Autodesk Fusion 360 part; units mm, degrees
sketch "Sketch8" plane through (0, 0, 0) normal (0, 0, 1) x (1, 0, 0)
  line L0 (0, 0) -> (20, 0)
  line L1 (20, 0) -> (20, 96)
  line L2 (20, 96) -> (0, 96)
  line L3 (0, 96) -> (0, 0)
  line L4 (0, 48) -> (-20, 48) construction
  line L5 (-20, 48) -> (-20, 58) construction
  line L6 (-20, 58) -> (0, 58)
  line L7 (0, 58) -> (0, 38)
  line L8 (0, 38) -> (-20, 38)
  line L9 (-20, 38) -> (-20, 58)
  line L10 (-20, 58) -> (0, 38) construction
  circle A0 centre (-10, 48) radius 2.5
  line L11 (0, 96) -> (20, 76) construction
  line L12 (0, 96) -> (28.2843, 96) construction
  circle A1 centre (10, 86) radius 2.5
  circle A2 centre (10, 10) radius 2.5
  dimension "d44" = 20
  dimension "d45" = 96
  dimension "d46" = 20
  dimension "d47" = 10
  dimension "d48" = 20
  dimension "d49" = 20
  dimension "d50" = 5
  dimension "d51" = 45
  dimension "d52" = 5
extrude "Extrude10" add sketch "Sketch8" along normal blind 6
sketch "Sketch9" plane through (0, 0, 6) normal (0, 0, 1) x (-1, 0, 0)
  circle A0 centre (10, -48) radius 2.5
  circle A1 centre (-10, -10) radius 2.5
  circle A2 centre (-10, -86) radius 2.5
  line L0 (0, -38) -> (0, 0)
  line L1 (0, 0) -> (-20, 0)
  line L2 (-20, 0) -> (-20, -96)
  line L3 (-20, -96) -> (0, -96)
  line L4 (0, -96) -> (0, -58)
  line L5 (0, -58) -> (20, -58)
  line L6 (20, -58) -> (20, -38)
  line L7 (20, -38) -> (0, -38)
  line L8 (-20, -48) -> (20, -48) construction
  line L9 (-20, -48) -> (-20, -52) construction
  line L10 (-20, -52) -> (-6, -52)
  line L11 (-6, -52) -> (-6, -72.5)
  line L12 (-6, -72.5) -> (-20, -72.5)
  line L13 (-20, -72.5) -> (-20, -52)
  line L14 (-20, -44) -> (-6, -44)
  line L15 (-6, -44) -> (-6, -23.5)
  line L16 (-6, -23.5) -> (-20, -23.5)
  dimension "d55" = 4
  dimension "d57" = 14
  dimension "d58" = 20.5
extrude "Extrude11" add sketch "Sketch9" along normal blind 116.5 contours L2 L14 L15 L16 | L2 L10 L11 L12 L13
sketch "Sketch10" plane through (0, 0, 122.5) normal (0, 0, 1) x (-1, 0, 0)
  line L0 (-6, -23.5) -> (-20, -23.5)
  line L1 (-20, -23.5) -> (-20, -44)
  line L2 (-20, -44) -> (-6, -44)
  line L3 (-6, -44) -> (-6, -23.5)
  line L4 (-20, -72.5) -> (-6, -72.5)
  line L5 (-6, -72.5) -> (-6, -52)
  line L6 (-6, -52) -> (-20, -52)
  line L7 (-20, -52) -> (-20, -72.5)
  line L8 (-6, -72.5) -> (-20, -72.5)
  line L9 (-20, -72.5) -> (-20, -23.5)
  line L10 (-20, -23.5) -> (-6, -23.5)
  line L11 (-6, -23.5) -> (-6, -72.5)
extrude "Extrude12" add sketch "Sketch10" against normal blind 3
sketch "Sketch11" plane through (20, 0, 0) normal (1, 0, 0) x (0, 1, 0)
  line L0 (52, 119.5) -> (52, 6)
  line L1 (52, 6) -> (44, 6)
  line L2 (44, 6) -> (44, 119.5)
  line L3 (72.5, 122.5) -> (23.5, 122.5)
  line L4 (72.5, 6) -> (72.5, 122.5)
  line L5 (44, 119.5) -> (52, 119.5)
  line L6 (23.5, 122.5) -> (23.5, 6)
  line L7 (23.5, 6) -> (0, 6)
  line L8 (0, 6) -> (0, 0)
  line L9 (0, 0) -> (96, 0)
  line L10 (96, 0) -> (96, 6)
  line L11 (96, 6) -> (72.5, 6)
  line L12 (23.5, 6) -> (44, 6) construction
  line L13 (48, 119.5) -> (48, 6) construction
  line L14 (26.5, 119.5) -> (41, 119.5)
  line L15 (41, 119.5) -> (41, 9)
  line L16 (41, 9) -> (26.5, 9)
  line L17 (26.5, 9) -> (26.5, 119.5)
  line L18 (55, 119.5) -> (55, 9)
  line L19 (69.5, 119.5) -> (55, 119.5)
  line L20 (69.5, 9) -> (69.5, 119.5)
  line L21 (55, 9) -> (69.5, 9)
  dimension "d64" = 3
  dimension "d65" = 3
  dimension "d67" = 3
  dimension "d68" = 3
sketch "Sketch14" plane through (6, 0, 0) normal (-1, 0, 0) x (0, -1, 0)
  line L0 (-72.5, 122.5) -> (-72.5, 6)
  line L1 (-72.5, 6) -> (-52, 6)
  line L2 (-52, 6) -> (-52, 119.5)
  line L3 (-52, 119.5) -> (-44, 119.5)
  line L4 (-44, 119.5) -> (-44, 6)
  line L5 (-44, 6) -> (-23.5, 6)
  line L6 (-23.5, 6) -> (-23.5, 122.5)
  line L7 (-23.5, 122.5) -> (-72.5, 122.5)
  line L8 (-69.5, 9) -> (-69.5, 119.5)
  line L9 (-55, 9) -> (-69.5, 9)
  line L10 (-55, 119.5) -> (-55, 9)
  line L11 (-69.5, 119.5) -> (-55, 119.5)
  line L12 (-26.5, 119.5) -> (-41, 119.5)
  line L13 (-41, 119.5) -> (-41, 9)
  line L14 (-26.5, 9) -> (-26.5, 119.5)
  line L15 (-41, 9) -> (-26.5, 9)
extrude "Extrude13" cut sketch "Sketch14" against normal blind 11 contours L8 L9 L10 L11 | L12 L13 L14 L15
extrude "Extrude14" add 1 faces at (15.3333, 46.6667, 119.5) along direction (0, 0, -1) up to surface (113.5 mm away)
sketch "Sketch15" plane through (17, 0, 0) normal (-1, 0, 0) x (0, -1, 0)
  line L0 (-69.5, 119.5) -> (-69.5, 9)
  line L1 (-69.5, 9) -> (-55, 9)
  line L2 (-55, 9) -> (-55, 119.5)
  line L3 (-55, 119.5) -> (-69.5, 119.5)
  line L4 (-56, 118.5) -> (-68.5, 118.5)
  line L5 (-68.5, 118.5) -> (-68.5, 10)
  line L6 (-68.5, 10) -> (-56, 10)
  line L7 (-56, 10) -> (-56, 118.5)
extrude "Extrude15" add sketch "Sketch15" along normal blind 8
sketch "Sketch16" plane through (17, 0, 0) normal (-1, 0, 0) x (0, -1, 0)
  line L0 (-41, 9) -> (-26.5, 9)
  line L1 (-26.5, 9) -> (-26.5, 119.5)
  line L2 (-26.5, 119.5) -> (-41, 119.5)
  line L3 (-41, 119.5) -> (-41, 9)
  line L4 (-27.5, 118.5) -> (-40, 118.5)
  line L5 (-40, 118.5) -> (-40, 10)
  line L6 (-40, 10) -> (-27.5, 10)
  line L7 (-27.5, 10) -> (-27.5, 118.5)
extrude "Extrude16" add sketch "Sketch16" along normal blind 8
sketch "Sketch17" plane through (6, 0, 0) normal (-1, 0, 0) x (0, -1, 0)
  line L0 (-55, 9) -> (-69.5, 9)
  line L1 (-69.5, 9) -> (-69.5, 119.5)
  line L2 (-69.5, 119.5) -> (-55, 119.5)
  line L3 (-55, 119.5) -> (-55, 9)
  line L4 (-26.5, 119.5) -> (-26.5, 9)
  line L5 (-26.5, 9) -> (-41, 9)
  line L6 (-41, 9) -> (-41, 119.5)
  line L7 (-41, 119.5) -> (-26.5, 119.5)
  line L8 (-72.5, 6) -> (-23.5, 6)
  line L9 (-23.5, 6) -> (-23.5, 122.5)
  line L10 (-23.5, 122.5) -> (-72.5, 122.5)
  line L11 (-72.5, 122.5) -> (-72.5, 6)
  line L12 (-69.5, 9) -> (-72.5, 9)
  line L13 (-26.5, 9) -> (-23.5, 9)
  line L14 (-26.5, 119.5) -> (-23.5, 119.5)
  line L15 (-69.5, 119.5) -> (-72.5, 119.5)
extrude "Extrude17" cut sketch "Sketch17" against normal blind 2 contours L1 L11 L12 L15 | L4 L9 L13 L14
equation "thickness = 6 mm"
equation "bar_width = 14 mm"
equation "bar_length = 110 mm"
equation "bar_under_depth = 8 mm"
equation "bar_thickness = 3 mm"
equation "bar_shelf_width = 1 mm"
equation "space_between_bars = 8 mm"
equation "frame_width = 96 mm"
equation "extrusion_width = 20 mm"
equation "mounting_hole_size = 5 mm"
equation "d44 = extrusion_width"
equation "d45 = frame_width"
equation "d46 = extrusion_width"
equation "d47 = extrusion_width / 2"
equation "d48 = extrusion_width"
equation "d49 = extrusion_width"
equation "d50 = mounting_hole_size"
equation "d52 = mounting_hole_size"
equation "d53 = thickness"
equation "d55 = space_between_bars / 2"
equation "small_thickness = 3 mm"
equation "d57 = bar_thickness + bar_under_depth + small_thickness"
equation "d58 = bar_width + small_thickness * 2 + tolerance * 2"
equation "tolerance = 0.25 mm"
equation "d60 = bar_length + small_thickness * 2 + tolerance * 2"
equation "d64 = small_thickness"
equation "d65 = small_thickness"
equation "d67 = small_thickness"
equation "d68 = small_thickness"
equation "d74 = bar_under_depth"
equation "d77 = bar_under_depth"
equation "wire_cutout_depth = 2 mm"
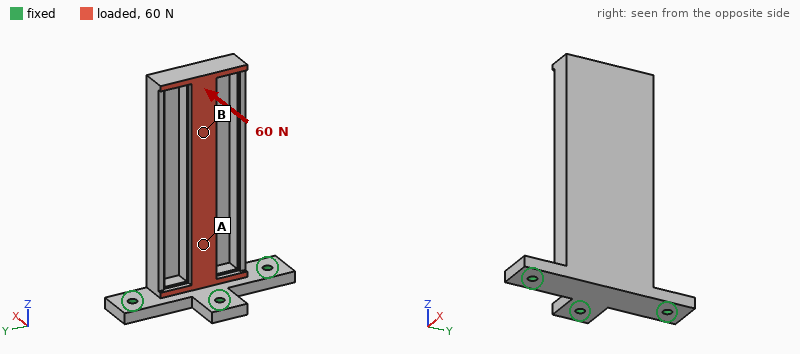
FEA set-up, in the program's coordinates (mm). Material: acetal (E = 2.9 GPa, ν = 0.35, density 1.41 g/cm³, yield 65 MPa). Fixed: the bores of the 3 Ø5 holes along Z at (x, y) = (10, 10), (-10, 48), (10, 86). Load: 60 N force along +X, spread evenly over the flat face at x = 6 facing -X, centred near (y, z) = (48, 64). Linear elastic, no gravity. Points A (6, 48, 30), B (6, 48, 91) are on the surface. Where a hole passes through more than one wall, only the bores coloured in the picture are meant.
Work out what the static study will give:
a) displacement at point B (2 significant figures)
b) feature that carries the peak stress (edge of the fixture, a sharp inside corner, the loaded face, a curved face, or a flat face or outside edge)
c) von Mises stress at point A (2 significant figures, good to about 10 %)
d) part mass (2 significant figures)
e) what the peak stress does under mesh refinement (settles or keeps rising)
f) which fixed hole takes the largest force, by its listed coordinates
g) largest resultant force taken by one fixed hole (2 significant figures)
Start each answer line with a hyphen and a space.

- 1.2 mm
- edge of the fixture
- 3.1 MPa
- 86 g
- keeps rising
- (-10, 48)
- 150 N
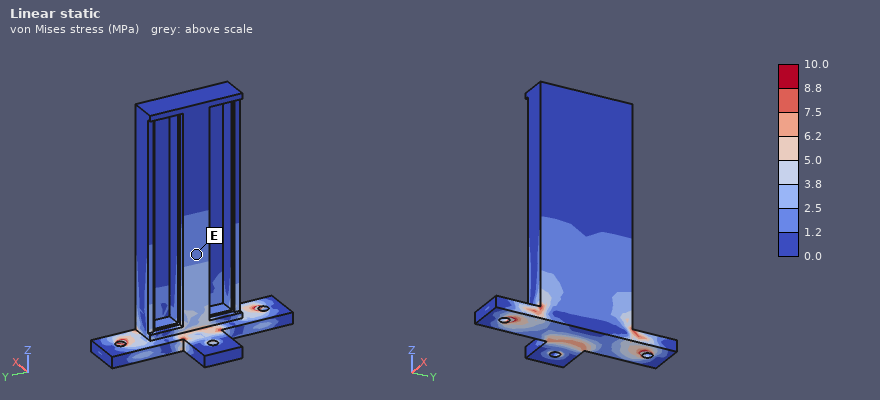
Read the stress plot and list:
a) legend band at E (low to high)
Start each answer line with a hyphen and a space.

- 1.2 to 2.5 MPa
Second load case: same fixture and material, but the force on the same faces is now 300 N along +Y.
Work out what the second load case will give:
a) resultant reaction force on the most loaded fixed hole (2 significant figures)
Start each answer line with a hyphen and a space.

- 320 N
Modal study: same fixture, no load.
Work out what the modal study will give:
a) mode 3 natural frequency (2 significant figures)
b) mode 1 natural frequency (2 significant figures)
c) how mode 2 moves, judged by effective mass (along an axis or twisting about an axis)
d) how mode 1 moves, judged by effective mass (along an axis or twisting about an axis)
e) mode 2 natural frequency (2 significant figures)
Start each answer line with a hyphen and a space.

- 680 Hz
- 140 Hz
- along Y
- along X
- 360 Hz
